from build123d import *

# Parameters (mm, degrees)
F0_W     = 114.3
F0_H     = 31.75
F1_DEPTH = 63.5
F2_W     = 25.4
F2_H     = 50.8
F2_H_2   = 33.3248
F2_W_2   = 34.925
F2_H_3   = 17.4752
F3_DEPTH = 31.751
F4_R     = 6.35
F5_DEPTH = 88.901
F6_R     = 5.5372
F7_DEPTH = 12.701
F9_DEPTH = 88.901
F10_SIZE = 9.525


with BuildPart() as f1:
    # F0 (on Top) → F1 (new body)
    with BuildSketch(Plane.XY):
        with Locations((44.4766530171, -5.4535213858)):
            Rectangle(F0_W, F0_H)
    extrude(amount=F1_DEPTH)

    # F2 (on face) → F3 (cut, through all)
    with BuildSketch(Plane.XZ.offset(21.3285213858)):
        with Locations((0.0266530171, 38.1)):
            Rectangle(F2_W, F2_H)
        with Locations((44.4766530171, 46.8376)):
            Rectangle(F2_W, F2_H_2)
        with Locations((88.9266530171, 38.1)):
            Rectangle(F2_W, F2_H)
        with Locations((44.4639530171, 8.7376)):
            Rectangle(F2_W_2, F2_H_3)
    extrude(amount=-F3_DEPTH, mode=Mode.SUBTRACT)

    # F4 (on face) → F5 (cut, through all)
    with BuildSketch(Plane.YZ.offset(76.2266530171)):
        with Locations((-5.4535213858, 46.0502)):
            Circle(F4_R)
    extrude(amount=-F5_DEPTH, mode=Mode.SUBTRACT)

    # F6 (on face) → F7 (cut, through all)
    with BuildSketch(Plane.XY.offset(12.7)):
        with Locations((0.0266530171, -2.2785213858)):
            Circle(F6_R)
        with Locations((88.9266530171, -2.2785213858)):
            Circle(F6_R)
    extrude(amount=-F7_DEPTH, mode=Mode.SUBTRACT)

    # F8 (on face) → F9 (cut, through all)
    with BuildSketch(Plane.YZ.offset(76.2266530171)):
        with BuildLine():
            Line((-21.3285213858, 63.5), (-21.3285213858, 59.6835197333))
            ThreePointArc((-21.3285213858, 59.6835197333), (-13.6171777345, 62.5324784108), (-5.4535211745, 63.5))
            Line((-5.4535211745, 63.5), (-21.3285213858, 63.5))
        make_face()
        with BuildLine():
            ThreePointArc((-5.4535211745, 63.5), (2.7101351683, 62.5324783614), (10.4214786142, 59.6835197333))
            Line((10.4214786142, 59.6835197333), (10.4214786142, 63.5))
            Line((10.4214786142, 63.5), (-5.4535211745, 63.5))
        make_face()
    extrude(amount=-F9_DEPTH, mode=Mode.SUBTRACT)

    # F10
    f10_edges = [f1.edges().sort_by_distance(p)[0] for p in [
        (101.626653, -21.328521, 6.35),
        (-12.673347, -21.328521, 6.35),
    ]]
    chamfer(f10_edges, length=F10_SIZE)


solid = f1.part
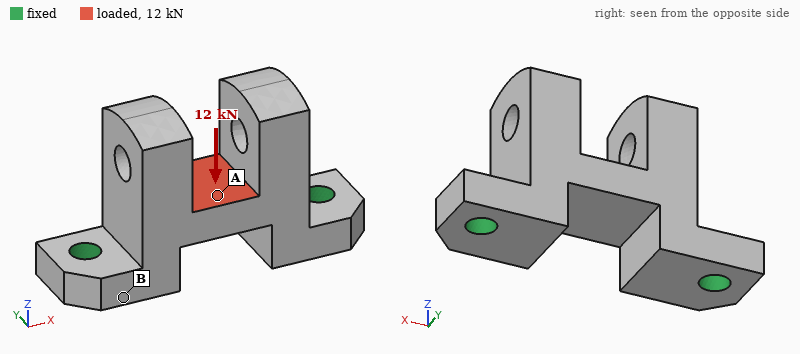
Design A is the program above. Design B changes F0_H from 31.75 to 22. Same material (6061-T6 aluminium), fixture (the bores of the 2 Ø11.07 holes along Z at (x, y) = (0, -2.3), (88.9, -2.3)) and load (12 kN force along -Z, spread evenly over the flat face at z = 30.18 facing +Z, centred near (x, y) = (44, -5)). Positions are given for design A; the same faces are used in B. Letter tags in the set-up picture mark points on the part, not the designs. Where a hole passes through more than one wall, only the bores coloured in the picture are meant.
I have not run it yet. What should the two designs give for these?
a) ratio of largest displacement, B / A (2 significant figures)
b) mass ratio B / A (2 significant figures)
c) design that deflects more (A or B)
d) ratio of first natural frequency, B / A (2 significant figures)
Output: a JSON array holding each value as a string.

["1.3", "0.67", "B", "0.93"]
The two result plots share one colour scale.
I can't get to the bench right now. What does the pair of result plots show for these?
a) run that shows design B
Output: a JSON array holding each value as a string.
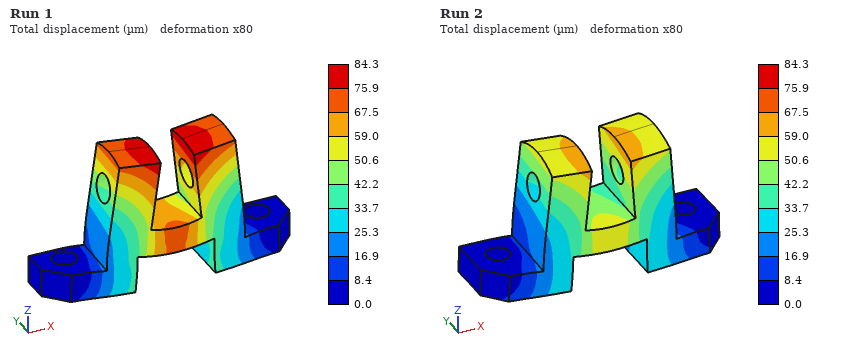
["Run 1"]
